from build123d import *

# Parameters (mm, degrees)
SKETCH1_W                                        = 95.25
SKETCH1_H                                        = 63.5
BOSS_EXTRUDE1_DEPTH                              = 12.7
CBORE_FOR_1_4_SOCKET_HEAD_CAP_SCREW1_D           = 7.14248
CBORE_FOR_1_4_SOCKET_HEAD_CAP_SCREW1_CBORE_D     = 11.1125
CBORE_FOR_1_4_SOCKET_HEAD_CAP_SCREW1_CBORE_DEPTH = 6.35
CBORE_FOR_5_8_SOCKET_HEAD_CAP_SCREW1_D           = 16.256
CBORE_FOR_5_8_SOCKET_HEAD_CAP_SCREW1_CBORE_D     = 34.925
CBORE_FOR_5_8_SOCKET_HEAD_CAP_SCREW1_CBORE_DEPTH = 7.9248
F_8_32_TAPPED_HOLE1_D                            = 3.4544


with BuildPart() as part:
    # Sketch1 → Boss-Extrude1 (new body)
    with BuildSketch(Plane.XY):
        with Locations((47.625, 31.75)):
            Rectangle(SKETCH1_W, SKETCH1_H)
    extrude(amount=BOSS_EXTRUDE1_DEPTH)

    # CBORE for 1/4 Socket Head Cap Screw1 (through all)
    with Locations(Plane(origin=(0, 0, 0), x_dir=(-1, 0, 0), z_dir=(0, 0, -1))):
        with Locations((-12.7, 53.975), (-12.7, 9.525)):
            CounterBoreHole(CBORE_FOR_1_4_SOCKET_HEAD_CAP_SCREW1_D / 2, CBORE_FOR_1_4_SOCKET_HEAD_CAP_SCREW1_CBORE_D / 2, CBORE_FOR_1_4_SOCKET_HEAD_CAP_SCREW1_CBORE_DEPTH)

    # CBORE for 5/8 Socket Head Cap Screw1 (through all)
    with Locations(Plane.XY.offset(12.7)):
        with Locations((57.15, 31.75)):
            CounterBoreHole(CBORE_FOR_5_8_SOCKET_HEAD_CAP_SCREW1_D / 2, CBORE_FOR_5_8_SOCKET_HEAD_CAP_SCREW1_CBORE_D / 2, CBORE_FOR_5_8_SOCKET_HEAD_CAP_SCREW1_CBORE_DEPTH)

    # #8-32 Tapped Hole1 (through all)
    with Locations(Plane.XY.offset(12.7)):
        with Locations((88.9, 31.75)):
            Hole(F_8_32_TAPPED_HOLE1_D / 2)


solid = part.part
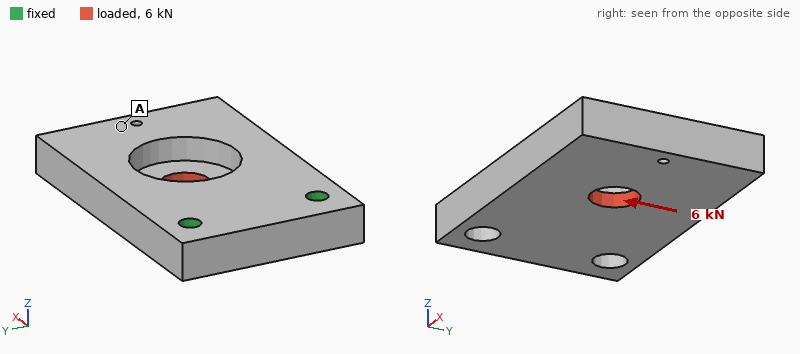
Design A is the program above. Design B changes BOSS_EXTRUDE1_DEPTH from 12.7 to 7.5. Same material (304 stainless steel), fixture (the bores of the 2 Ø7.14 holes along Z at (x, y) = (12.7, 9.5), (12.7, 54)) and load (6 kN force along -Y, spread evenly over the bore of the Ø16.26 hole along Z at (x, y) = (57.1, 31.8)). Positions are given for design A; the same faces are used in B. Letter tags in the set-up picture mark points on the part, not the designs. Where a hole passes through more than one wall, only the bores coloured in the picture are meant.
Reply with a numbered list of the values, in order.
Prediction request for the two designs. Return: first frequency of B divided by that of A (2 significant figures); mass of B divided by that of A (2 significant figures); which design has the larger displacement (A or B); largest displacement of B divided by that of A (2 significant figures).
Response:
1. 0.43
2. 0.61
3. B
4. 2.7
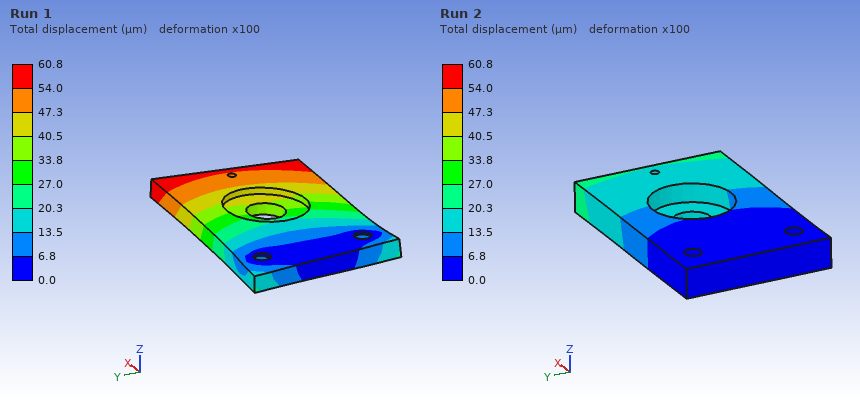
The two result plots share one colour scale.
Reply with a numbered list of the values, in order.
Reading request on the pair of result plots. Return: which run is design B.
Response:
1. Run 1
